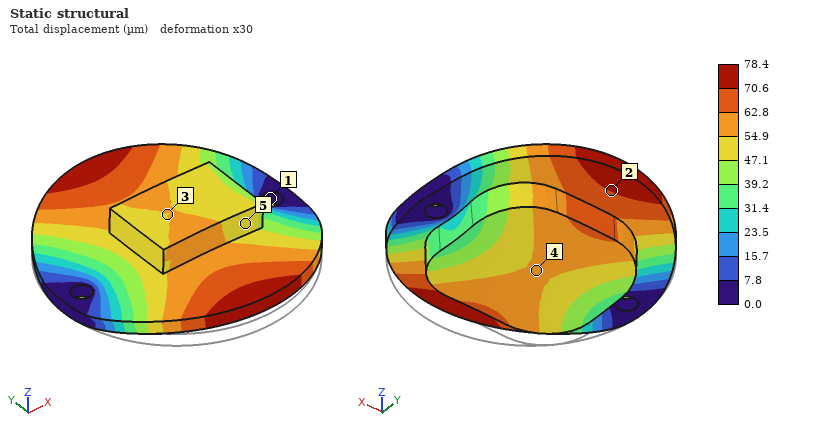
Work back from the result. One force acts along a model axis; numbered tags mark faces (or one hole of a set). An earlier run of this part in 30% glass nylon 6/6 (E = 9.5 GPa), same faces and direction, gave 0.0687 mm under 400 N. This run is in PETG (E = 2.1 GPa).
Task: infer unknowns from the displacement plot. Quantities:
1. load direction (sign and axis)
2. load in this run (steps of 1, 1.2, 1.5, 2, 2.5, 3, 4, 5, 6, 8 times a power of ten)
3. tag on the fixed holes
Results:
+Z
100 N
1
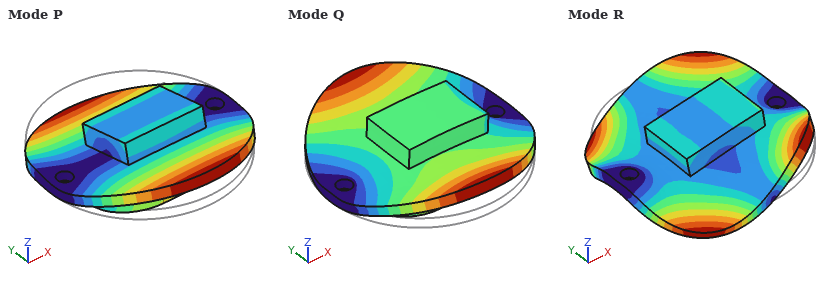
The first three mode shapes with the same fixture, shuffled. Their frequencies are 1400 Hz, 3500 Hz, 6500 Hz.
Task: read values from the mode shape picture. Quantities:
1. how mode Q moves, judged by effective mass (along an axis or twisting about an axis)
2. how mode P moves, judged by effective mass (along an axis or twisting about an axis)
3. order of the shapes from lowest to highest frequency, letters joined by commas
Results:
along Z
twisting about X
P, Q, R
